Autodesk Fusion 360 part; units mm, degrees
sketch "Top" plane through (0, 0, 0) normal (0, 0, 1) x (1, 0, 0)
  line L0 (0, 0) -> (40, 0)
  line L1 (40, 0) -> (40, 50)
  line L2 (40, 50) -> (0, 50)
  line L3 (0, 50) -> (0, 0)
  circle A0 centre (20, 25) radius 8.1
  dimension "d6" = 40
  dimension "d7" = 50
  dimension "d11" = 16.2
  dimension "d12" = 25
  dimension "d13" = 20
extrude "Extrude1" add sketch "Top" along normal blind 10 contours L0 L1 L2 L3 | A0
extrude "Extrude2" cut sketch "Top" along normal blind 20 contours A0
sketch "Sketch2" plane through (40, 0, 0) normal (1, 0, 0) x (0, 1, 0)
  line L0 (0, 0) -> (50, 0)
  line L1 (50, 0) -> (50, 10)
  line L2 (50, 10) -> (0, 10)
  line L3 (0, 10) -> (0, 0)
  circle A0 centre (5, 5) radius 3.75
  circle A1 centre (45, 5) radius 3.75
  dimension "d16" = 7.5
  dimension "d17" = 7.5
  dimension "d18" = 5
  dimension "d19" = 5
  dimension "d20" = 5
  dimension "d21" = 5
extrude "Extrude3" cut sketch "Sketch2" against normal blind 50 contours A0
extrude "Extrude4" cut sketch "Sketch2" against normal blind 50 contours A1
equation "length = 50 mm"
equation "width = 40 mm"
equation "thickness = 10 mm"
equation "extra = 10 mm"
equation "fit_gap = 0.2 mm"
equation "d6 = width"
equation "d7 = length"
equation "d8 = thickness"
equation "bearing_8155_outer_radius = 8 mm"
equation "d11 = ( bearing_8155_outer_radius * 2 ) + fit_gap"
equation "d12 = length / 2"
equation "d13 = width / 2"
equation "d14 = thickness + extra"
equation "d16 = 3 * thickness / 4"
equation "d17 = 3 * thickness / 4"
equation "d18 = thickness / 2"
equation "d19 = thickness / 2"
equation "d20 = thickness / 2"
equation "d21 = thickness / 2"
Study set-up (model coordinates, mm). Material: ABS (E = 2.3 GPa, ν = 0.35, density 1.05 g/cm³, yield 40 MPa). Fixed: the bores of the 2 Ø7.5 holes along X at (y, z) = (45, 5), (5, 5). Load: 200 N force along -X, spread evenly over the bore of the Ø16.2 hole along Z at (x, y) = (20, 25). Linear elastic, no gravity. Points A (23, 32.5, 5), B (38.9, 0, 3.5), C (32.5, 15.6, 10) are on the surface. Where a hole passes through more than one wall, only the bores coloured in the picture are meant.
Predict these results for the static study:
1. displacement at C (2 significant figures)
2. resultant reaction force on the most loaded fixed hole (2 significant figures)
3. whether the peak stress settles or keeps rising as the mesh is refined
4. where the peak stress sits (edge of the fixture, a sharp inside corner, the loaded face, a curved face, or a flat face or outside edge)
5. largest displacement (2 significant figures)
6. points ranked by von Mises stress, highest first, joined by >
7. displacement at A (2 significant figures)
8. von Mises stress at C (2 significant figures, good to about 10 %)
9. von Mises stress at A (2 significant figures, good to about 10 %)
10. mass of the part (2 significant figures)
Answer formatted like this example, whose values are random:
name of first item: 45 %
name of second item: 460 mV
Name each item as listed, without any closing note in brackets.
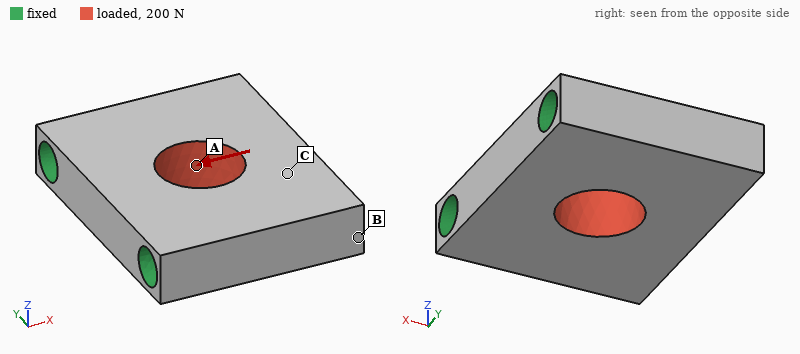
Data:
displacement at C: 2.5 µm
resultant reaction force on the most loaded fixed hole: 100 N
whether the peak stress settles or keeps rising as the mesh is refined: keeps rising
where the peak stress sits: edge of the fixture
largest displacement: 5.3 µm
points ranked by von Mises stress, highest first, joined by >: A > C > B
displacement at A: 3.5 µm
von Mises stress at C: 0.46 MPa
von Mises stress at A: 0.77 MPa
mass of the part: 15 g
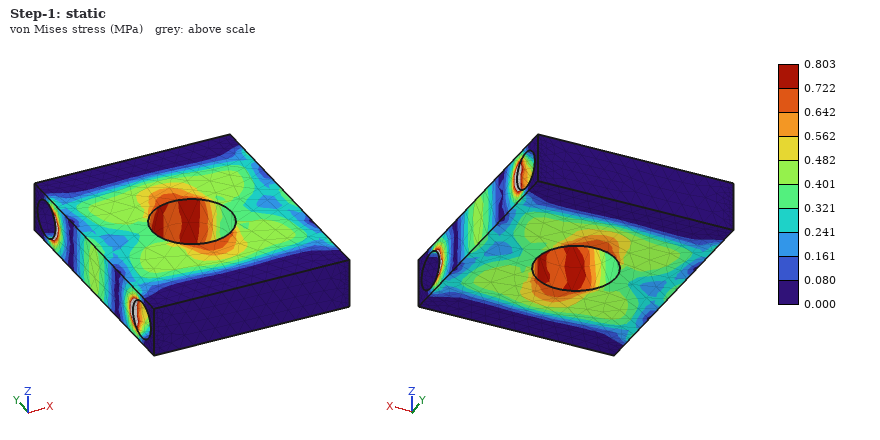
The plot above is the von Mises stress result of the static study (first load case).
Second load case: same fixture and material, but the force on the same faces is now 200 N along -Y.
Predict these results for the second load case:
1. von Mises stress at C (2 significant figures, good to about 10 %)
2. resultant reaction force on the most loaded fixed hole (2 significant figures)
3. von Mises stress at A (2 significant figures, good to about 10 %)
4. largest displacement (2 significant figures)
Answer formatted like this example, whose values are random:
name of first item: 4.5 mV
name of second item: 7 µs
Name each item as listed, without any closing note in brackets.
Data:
von Mises stress at C: 0.21 MPa
resultant reaction force on the most loaded fixed hole: 100 N
von Mises stress at A: 0.42 MPa
largest displacement: 2.3 µm
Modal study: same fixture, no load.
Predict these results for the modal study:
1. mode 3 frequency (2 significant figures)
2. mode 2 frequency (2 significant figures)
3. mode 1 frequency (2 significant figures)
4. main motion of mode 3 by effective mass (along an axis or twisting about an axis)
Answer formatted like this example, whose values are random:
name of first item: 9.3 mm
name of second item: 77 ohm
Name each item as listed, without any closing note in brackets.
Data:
mode 3 frequency: 13 kHz
mode 2 frequency: 9200 Hz
mode 1 frequency: 9000 Hz
main motion of mode 3 by effective mass: along X
